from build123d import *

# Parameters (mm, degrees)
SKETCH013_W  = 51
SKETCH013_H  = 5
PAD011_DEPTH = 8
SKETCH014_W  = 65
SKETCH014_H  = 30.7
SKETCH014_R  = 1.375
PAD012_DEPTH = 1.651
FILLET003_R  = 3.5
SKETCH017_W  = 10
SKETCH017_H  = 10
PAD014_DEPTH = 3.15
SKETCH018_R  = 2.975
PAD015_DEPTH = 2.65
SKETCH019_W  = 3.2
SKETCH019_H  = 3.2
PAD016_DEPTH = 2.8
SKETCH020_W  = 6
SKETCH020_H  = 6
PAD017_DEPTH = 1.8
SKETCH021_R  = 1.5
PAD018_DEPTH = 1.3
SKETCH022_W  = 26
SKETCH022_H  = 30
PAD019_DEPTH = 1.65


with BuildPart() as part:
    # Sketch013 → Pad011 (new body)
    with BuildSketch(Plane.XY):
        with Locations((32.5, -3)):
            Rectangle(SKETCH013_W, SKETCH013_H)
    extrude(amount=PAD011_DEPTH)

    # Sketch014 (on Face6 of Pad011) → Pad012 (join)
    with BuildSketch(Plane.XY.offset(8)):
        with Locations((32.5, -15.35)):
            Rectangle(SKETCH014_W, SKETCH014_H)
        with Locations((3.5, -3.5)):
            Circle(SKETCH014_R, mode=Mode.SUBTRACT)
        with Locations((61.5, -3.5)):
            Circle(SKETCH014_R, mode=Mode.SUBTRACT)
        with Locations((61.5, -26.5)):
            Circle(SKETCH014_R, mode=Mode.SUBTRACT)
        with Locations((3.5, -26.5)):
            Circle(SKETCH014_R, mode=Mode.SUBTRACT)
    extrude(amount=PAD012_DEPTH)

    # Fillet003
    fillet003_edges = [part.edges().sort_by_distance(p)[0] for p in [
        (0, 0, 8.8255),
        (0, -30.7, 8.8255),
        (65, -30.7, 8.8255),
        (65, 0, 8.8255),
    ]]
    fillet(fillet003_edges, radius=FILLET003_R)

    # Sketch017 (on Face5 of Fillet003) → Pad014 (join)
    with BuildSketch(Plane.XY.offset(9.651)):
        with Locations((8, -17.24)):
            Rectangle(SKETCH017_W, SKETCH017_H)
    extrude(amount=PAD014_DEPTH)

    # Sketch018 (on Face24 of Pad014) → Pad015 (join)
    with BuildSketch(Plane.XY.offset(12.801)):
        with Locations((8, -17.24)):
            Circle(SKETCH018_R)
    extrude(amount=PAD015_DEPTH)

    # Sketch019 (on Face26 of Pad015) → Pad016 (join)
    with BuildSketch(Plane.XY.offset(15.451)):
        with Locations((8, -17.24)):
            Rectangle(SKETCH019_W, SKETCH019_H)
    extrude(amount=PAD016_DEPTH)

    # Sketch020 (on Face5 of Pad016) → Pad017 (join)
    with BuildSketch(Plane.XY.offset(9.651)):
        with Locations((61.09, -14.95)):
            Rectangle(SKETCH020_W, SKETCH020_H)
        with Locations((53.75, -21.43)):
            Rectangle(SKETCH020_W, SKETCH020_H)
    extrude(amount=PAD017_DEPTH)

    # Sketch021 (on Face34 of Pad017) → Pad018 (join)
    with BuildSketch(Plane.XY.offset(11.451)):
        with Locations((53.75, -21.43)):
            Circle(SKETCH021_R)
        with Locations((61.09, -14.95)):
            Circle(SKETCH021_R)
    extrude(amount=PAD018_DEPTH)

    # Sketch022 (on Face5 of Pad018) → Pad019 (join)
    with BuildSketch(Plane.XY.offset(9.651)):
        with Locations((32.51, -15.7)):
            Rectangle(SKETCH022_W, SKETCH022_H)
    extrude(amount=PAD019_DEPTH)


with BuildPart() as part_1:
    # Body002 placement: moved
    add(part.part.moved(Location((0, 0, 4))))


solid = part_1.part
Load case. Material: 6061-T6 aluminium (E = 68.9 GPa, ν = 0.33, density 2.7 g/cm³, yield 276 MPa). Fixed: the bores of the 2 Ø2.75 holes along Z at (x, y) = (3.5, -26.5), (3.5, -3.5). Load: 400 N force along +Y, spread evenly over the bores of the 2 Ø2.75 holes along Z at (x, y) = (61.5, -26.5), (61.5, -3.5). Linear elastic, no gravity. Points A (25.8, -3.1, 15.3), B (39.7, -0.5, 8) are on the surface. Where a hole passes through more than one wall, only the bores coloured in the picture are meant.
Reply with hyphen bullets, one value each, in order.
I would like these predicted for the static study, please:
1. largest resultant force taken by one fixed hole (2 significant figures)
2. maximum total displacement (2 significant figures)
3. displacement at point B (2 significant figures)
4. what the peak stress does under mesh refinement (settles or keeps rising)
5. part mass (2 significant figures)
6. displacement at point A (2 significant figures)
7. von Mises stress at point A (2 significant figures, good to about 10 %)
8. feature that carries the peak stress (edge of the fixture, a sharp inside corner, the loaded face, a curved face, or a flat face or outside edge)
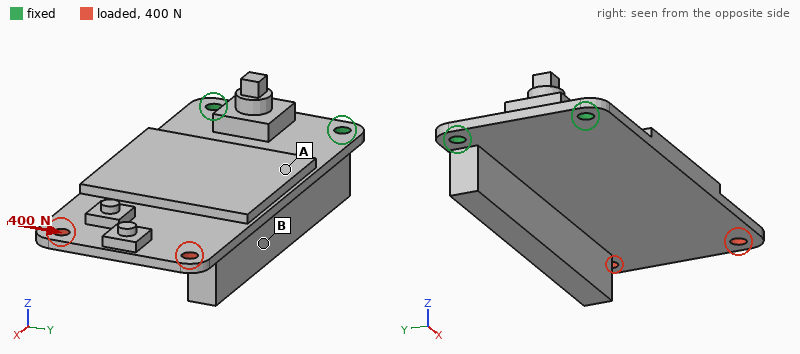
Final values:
- 1000 N
- 0.16 mm
- 0.077 mm
- keeps rising
- 19 g
- 0.037 mm
- 20 MPa
- edge of the fixture
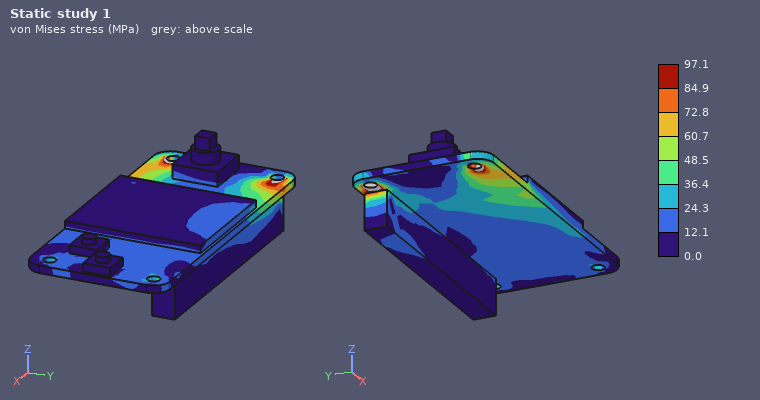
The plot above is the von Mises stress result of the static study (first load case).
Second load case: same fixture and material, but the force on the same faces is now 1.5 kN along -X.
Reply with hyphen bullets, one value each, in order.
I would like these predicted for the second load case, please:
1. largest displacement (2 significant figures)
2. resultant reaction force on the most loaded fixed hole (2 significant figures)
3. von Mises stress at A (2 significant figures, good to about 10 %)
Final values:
- 46 µm
- 760 N
- 12 MPa
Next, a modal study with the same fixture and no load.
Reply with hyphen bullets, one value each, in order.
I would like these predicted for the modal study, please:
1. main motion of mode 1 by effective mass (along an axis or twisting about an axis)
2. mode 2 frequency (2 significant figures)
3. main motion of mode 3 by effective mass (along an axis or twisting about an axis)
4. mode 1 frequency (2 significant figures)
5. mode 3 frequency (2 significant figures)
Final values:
- along Z
- 2300 Hz
- along Y
- 430 Hz
- 4400 Hz
